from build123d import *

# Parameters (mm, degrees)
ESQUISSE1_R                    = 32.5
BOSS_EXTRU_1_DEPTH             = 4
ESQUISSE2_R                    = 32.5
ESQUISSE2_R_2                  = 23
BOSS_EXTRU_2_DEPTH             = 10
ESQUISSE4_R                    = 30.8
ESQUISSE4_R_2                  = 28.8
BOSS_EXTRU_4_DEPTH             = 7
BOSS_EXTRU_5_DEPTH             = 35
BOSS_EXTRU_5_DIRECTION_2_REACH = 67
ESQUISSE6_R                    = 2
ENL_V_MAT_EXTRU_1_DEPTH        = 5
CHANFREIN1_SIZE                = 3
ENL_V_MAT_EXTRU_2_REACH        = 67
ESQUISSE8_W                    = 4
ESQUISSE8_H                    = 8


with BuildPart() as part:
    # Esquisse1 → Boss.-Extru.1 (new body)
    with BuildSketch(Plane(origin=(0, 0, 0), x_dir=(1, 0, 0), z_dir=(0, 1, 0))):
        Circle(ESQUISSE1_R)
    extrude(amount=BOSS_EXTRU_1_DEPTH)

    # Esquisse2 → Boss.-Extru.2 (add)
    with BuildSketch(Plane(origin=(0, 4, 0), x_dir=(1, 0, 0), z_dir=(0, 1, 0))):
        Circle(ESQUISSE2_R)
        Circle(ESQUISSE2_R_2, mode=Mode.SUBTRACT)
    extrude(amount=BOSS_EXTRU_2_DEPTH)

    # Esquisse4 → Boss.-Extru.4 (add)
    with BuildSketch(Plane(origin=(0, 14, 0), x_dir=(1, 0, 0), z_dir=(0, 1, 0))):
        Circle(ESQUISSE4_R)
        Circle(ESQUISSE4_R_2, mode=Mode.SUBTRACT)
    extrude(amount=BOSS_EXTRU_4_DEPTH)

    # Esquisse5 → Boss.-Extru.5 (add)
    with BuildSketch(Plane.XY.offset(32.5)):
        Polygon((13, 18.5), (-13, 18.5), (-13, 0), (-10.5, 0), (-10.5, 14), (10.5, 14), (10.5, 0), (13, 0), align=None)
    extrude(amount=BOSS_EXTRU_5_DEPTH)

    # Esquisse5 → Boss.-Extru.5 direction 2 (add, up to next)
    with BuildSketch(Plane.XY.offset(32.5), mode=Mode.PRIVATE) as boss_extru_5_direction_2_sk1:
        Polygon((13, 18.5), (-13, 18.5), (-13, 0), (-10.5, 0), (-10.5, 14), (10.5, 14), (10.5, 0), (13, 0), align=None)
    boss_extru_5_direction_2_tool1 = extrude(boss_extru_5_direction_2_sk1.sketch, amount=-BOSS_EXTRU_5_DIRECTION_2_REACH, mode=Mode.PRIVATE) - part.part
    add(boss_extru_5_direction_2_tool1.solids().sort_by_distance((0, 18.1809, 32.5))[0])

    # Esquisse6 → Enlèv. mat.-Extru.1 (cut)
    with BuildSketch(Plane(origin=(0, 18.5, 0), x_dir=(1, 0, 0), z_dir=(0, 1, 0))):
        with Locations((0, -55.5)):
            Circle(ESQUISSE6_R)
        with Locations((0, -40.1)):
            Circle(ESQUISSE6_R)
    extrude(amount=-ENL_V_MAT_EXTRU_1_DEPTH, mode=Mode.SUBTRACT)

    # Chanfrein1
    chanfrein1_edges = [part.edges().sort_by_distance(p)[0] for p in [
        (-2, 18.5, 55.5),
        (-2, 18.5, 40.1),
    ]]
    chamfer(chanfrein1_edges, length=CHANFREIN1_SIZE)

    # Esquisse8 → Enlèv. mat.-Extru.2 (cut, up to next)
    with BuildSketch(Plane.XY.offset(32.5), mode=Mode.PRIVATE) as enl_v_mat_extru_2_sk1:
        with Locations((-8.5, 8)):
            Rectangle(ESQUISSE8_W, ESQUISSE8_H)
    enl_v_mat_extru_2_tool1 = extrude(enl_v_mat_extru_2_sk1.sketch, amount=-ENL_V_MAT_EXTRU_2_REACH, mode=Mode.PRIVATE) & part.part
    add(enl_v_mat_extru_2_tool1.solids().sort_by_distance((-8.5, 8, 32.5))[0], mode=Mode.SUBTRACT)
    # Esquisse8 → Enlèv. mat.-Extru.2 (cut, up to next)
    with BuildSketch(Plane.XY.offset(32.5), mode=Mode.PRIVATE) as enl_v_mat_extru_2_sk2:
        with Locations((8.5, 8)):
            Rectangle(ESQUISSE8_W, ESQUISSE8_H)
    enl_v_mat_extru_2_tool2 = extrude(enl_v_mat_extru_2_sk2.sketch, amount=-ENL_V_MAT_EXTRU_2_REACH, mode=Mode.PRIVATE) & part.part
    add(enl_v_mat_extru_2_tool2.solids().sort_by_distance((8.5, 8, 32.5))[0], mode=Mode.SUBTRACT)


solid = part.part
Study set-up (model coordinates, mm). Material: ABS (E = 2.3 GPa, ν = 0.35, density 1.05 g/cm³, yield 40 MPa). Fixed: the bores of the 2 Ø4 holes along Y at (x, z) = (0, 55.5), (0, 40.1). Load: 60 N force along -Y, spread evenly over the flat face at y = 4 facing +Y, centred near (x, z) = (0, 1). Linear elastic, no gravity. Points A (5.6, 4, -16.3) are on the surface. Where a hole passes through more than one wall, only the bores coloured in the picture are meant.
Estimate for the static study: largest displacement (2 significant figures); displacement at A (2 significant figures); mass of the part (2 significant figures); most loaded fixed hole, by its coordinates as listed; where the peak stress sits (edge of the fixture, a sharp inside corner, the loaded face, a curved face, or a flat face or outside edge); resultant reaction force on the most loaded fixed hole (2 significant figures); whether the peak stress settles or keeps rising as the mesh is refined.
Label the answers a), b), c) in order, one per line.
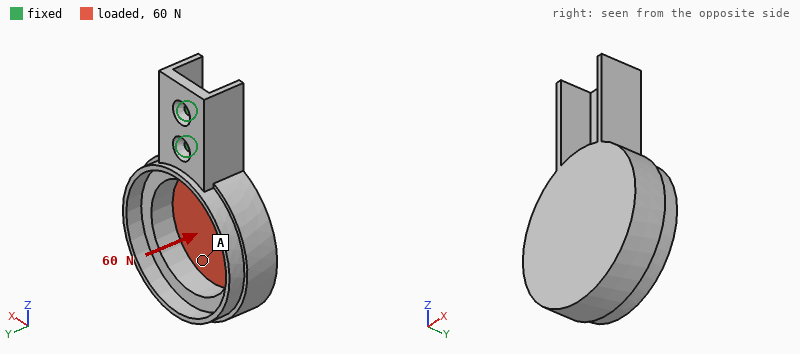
a) 1.2 mm
b) 0.91 mm
c) 40 g
d) (0, 40.1)
e) edge of the fixture
f) 180 N
g) keeps rising
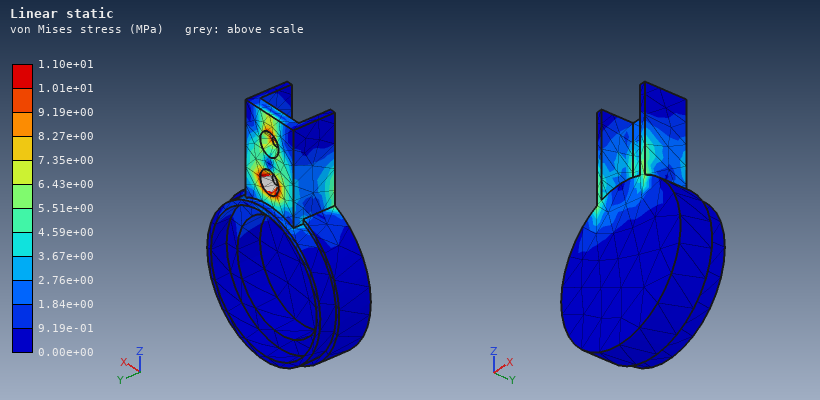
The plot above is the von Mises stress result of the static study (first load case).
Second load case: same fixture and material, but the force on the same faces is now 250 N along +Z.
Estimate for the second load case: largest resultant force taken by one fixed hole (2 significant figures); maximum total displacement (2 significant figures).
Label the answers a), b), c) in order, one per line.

a) 200 N
b) 1.1 mm
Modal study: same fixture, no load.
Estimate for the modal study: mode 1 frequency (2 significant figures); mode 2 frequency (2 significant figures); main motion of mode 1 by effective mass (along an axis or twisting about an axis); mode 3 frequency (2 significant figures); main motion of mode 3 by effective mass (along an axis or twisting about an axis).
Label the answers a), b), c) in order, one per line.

a) 230 Hz
b) 270 Hz
c) along Y
d) 340 Hz
e) along X
